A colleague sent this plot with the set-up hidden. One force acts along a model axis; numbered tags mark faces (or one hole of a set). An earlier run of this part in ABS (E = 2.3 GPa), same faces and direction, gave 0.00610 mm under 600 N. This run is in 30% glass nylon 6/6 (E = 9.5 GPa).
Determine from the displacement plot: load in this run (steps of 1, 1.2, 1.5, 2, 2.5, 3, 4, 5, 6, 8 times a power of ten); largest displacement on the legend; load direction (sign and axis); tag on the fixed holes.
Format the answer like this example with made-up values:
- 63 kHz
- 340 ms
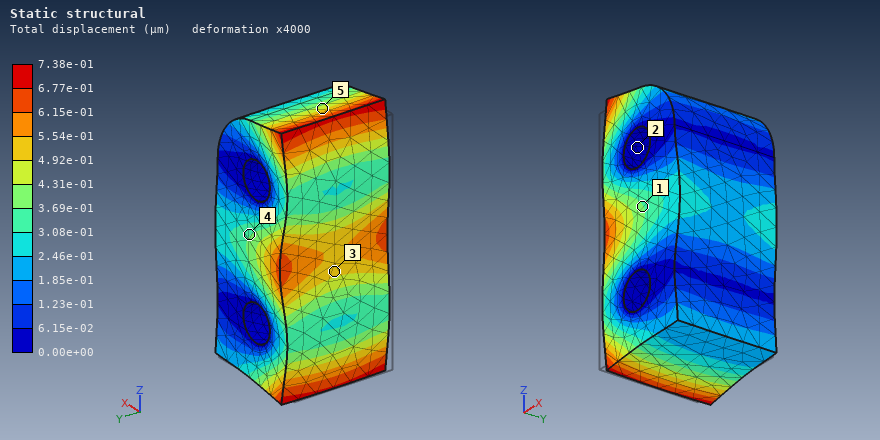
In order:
- 300 N
- 7.38e-01 µm
- +X
- 2
